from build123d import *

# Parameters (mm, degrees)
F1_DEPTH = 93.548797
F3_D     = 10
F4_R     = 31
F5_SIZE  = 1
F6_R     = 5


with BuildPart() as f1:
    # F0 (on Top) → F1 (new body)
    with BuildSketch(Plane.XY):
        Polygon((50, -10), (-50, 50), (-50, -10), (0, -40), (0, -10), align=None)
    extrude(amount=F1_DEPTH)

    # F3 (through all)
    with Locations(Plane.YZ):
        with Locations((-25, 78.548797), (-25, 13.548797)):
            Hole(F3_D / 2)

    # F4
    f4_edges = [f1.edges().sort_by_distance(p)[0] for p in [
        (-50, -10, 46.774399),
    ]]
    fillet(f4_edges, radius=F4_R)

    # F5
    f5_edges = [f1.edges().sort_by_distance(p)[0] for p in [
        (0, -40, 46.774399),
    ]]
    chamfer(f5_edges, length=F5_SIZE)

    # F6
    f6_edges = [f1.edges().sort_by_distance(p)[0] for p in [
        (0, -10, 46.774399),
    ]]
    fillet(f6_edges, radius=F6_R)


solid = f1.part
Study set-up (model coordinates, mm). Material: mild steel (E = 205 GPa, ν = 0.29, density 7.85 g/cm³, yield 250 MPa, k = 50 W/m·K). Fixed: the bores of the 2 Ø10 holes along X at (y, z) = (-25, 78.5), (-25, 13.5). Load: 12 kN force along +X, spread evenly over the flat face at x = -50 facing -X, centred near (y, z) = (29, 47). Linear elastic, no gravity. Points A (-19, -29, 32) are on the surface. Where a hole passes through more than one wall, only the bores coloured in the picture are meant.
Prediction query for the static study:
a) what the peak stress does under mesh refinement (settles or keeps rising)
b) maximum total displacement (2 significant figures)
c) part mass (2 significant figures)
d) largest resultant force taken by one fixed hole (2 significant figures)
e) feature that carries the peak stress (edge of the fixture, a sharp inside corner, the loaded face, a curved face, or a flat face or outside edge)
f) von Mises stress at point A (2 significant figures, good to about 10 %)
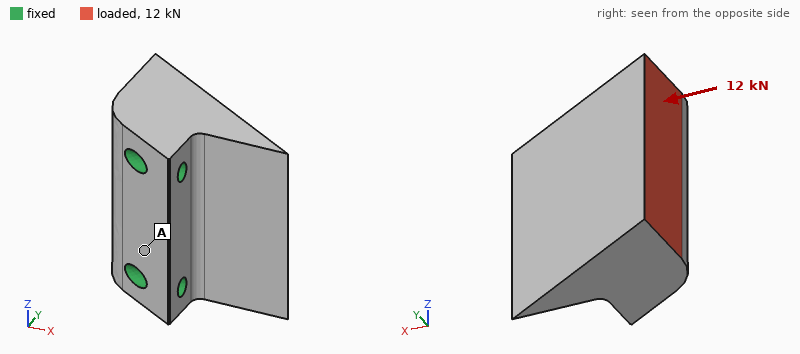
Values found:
keeps rising
29 µm
2.7 kg
6.1 kN
edge of the fixture
12 MPa
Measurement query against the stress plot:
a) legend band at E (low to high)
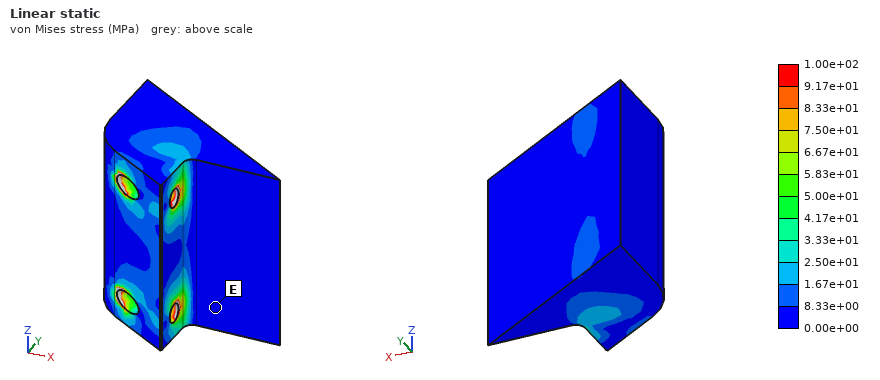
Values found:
0.00e+00 to 8.33e+00 MPa
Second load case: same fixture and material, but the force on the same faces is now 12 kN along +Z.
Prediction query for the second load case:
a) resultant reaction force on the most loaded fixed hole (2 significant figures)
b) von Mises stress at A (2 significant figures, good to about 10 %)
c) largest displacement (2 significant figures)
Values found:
12 kN
5.1 MPa
9.7 µm
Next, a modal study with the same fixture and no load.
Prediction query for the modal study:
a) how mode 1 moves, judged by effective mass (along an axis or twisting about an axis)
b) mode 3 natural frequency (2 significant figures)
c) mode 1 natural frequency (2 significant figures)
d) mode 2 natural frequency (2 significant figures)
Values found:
along X
7600 Hz
3500 Hz
7300 Hz
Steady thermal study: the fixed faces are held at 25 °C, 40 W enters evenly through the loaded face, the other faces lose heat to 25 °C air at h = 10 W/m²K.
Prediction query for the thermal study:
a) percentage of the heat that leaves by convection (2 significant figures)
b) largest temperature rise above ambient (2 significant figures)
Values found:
5.3 %
18 K
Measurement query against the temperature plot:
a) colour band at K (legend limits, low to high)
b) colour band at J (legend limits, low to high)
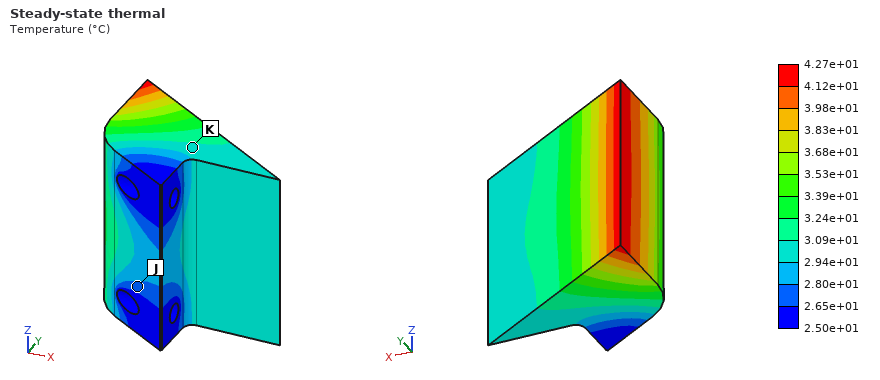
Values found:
2.94e+01 to 3.09e+01 °C
2.65e+01 to 2.80e+01 °C
